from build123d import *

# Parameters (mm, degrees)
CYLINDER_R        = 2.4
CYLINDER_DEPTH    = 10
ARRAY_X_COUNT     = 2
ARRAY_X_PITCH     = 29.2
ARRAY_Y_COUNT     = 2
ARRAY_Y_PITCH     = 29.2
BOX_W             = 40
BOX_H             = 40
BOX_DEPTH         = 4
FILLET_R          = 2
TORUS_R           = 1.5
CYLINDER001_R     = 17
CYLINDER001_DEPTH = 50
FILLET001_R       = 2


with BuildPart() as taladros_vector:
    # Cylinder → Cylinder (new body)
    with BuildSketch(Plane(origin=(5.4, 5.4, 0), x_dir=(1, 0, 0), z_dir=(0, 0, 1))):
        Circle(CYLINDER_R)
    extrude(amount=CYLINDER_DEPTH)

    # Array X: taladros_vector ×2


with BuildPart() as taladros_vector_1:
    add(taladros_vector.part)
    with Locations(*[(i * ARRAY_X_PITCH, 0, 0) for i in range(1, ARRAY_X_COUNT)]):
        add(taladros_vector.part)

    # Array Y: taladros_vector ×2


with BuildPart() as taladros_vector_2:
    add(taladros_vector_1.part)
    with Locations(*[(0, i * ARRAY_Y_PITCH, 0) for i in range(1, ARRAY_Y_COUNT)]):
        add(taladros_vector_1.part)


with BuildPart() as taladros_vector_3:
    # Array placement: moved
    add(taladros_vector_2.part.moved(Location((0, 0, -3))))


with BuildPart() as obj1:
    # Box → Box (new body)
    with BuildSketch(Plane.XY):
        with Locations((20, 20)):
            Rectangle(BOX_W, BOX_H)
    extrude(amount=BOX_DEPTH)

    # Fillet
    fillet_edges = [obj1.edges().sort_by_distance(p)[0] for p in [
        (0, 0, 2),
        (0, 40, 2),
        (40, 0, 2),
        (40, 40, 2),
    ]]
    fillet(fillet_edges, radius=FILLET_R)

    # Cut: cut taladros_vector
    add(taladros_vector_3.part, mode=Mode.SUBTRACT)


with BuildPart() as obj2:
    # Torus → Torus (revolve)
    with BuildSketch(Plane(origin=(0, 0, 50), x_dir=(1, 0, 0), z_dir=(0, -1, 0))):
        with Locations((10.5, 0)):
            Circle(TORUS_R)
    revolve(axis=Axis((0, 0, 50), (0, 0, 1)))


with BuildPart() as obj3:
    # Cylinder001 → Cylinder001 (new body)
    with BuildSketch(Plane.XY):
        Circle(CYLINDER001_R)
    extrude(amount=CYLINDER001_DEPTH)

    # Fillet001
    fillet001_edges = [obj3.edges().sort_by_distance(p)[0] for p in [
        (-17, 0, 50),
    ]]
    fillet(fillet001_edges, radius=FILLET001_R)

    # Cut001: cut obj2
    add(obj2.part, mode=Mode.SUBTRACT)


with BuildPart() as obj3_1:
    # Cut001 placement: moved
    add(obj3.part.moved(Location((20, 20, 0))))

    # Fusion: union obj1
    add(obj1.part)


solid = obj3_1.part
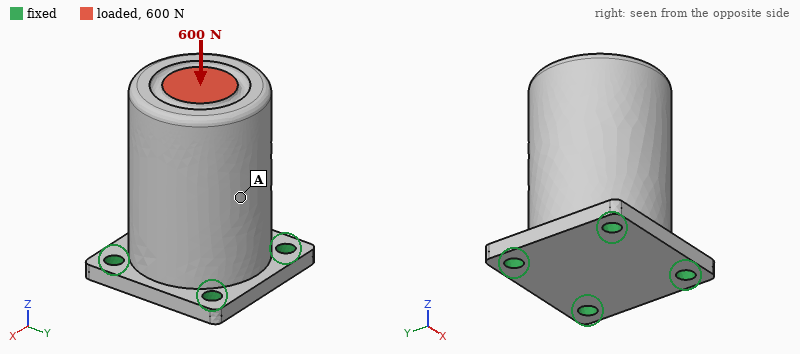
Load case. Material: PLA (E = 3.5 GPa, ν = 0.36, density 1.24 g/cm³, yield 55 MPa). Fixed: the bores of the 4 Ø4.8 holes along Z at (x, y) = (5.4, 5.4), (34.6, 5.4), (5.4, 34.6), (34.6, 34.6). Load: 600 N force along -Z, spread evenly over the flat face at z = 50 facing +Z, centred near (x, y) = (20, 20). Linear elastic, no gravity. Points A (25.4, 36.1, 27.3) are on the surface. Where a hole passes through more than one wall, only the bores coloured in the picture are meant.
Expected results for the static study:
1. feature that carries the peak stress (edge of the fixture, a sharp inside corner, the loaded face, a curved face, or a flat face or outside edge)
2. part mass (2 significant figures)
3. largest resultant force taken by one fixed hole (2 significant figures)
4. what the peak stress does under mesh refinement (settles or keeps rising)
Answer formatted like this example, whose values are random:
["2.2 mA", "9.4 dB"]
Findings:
["edge of the fixture", "59 g", "160 N", "keeps rising"]
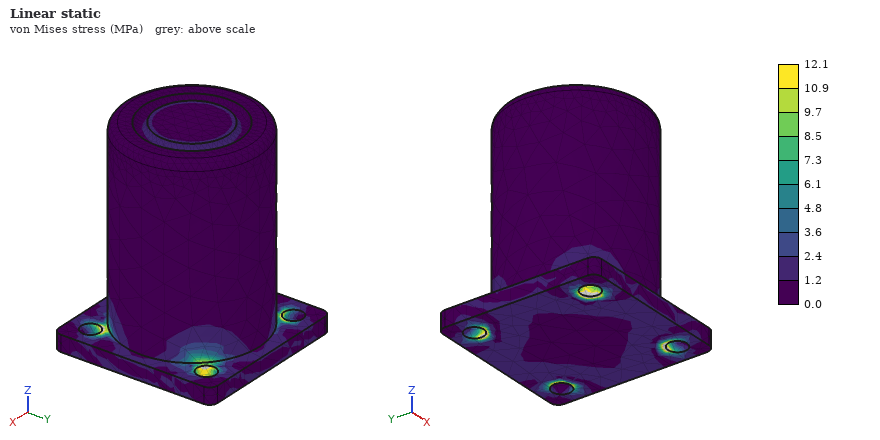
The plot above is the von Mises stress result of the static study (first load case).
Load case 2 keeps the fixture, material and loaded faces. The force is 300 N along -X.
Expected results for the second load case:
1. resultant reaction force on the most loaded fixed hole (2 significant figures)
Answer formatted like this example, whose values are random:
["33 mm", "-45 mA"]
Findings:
["300 N"]
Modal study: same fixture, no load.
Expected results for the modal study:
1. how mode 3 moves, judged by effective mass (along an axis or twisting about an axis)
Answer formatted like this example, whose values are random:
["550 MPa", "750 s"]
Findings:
["along Z"]
